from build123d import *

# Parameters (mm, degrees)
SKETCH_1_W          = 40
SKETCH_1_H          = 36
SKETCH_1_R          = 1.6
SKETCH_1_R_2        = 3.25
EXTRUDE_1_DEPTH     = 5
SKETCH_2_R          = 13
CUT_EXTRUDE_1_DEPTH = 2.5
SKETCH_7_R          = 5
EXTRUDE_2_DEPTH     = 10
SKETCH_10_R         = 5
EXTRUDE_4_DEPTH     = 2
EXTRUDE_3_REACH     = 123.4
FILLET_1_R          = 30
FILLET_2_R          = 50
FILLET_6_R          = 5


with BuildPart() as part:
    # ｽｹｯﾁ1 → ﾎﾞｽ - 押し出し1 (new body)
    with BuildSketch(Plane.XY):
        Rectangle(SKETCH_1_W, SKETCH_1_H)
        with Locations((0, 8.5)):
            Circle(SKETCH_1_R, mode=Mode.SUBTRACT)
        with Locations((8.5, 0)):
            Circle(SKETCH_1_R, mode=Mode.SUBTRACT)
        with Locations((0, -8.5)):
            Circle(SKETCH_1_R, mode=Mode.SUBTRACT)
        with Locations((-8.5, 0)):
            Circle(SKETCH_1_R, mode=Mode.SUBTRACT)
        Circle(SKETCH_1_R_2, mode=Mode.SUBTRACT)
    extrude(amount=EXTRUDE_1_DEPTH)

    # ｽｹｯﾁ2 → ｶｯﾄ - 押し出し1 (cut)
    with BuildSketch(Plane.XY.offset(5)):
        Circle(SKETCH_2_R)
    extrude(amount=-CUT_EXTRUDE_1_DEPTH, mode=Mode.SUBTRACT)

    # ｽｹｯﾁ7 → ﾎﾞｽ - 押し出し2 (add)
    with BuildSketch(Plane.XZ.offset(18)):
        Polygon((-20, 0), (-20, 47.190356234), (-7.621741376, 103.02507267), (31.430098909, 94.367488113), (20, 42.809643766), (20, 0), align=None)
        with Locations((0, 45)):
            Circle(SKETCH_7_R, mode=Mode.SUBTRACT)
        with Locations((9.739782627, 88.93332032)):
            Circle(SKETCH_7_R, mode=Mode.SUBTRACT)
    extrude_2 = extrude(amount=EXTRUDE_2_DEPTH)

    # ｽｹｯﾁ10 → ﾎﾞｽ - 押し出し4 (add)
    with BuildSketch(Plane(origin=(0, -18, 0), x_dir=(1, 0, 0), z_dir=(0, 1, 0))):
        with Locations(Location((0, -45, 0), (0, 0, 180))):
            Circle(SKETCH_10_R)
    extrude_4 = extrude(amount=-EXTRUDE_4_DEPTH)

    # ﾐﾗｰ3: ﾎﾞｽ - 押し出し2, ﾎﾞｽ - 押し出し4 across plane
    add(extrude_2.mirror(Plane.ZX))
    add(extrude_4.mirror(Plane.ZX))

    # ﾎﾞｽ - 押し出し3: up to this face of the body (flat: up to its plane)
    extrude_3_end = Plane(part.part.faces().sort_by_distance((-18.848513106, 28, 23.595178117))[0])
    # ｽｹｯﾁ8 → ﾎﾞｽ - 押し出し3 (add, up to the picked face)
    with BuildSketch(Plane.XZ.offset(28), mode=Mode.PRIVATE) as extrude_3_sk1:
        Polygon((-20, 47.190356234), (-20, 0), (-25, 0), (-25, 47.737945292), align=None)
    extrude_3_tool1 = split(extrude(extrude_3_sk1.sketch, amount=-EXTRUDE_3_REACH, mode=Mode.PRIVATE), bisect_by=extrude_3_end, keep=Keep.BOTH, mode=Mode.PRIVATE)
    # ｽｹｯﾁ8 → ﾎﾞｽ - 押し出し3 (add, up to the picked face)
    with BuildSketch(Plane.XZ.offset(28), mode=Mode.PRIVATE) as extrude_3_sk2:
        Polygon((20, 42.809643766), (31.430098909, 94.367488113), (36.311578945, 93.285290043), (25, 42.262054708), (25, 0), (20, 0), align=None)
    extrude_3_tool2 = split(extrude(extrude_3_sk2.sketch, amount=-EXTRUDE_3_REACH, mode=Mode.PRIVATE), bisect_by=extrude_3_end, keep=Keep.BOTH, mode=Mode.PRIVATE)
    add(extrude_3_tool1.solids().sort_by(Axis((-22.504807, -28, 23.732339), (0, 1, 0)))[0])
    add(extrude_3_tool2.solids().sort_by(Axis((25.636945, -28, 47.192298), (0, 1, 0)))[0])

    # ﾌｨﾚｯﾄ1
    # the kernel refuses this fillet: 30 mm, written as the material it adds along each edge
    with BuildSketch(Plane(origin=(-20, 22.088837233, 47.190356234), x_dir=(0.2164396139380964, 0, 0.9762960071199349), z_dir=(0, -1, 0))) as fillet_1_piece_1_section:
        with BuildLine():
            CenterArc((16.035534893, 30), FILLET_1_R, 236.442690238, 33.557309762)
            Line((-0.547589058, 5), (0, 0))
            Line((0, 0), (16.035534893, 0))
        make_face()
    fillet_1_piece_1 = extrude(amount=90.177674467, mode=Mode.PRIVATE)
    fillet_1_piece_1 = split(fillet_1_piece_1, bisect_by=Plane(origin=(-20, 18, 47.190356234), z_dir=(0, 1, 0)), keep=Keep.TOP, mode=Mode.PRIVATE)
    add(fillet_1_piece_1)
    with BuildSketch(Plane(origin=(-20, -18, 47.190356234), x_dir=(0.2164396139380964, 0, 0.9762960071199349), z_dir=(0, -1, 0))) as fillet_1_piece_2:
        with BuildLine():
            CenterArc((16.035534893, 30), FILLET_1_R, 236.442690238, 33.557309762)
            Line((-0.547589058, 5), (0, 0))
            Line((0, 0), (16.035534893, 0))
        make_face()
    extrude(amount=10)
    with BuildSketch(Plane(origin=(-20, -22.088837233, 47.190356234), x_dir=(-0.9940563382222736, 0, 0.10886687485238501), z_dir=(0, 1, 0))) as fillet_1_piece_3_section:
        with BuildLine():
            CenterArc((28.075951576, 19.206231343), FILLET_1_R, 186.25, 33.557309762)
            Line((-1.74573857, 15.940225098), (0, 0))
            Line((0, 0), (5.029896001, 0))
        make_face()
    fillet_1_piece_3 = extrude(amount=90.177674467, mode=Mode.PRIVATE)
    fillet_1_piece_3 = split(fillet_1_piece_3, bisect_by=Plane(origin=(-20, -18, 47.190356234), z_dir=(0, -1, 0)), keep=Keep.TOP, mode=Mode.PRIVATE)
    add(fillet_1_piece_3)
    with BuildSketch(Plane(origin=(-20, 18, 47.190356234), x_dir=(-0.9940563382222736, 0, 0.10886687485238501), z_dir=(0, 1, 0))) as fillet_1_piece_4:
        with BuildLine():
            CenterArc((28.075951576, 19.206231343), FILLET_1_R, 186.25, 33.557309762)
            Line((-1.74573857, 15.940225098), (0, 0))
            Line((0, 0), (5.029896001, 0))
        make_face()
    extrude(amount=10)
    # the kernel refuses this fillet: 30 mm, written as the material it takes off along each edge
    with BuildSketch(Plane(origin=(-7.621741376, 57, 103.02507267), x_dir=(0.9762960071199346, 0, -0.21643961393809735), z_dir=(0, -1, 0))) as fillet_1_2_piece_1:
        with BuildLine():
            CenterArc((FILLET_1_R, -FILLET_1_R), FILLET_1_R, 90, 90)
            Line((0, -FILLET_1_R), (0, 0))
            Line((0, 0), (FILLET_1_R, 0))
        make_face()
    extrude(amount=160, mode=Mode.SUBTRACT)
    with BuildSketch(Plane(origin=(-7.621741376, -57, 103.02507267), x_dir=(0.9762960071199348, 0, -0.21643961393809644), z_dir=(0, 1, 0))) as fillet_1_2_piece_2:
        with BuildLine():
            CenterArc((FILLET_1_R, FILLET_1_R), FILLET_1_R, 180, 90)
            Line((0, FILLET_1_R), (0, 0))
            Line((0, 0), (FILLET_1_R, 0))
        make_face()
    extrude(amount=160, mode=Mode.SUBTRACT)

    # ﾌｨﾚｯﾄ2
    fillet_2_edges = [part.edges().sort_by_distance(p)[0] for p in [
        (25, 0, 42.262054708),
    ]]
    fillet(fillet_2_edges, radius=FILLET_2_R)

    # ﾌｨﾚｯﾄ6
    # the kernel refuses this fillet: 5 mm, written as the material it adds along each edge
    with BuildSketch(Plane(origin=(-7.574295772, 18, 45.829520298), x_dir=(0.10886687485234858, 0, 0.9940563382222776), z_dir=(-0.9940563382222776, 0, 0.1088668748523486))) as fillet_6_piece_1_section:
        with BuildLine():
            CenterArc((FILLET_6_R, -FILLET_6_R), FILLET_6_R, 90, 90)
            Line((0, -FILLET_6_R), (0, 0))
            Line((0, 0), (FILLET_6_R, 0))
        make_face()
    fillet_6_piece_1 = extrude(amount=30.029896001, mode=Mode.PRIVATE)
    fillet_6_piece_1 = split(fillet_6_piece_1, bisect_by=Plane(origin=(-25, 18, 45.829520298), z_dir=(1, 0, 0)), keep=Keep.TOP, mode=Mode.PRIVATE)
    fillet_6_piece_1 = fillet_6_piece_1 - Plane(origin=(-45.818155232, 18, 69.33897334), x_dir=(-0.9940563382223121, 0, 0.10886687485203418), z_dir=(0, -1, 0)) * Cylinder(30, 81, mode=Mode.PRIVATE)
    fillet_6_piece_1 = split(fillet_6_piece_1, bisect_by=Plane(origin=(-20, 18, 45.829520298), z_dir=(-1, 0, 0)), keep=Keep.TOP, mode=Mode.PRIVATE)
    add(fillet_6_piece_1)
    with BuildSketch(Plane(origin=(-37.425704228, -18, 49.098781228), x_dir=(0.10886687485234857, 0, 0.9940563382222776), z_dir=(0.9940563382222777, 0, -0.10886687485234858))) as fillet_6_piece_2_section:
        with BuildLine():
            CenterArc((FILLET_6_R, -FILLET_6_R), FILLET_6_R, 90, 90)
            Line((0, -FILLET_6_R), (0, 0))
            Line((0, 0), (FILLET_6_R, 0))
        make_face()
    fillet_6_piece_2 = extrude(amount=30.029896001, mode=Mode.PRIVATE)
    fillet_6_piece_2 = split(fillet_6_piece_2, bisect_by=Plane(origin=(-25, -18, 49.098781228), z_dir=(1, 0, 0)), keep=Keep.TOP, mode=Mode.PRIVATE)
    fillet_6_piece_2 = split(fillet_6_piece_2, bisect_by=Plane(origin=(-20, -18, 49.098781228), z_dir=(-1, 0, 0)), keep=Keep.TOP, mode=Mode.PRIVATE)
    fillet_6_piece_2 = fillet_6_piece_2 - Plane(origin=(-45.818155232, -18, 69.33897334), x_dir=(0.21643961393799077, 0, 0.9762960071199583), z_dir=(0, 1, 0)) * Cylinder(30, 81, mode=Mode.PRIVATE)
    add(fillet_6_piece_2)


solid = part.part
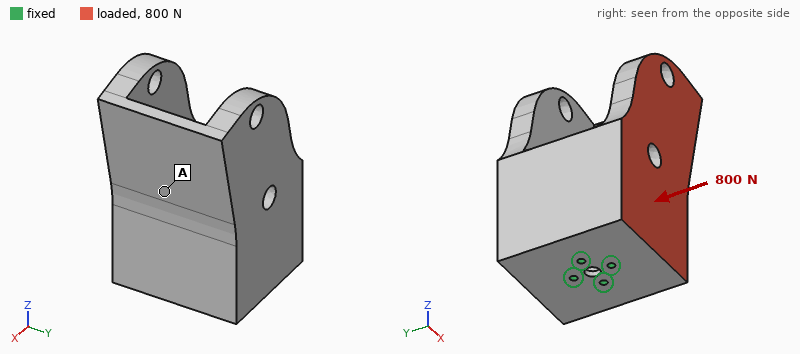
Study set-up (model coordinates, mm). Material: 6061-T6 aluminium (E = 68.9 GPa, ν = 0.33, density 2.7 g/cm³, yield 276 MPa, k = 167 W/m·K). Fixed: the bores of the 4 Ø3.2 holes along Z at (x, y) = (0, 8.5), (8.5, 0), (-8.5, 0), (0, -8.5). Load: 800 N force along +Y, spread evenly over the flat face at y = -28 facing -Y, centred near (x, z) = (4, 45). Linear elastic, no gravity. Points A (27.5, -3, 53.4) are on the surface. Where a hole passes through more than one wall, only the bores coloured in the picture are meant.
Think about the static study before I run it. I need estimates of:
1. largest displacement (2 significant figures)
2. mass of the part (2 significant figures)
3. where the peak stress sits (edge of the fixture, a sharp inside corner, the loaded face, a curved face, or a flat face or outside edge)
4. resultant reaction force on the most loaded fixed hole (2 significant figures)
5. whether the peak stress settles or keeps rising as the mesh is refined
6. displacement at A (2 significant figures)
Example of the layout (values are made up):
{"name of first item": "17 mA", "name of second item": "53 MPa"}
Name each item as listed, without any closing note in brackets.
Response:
{"largest displacement": "0.38 mm", "mass of the part": "320 g", "where the peak stress sits": "edge of the fixture", "resultant reaction force on the most loaded fixed hole": "1.4 kN", "whether the peak stress settles or keeps rising as the mesh is refined": "keeps rising", "displacement at A": "0.20 mm"}
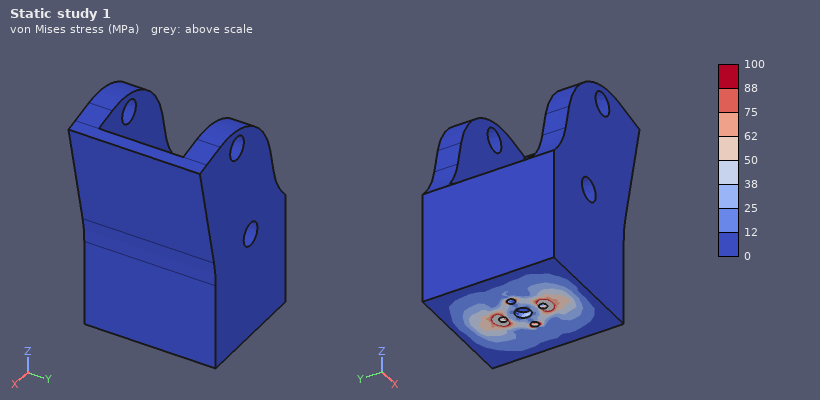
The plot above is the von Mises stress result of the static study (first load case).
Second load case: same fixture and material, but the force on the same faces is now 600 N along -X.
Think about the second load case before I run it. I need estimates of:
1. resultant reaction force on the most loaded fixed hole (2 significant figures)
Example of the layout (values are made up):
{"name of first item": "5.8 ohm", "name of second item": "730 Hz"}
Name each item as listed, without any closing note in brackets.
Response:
{"resultant reaction force on the most loaded fixed hole": "1.1 kN"}
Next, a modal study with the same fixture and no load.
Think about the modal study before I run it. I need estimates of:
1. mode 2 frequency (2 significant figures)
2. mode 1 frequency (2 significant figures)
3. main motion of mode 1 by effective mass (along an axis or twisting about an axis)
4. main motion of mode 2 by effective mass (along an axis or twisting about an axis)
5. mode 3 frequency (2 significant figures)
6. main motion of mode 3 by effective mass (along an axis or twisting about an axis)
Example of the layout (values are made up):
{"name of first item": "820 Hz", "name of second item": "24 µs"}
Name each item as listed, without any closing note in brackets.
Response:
{"mode 2 frequency": "510 Hz", "mode 1 frequency": "490 Hz", "main motion of mode 1 by effective mass": "along X", "main motion of mode 2 by effective mass": "along Y", "mode 3 frequency": "2700 Hz", "main motion of mode 3 by effective mass": "twisting about Z"}
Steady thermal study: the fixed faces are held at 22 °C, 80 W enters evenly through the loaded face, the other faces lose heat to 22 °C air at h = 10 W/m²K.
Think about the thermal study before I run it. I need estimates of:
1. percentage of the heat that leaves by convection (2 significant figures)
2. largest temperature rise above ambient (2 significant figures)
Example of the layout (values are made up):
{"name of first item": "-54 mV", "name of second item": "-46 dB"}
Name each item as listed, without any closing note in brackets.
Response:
{"percentage of the heat that leaves by convection": "11 %", "largest temperature rise above ambient": "47 K"}
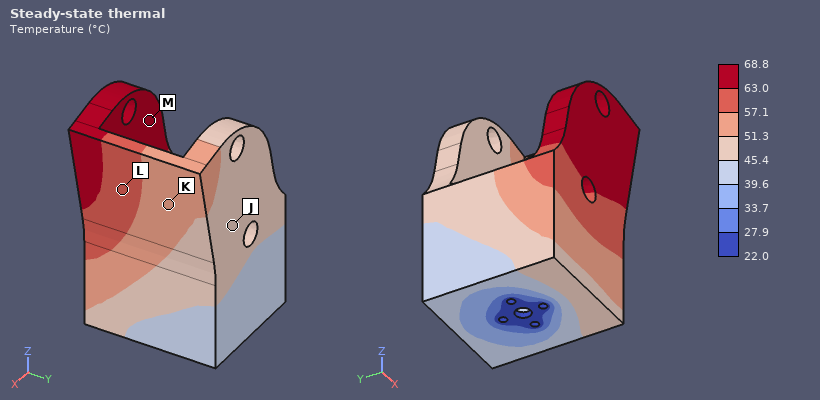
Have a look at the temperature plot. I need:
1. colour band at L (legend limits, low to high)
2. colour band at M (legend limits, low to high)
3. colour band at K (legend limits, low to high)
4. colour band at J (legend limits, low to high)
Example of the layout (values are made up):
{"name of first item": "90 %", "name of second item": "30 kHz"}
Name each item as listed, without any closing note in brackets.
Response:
{"colour band at L": "57.1 to 63.0 °C", "colour band at M": "63.0 to 68.8 °C", "colour band at K": "51.3 to 57.1 °C", "colour band at J": "45.4 to 51.3 °C"}
